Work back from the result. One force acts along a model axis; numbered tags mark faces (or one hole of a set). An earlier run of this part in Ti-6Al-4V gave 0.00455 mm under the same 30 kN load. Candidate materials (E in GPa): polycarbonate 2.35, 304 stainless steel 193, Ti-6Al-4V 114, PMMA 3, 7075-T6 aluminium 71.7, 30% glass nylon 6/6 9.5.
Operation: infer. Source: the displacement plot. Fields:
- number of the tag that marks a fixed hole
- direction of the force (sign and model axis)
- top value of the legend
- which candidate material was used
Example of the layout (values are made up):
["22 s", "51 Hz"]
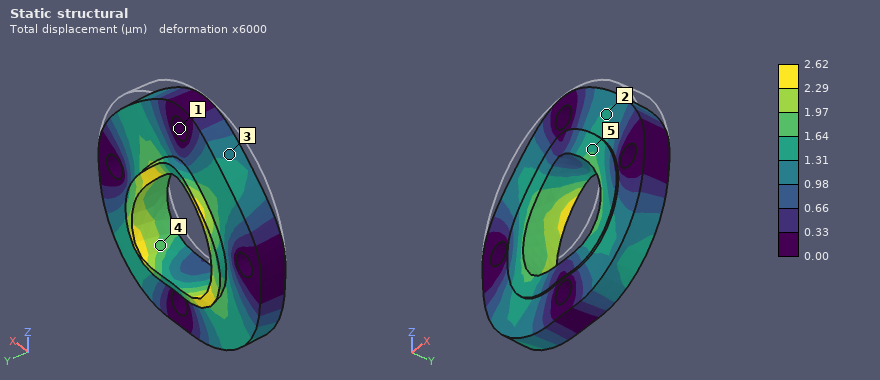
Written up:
["1", "-Z", "2.62 µm", "304 stainless steel"]
